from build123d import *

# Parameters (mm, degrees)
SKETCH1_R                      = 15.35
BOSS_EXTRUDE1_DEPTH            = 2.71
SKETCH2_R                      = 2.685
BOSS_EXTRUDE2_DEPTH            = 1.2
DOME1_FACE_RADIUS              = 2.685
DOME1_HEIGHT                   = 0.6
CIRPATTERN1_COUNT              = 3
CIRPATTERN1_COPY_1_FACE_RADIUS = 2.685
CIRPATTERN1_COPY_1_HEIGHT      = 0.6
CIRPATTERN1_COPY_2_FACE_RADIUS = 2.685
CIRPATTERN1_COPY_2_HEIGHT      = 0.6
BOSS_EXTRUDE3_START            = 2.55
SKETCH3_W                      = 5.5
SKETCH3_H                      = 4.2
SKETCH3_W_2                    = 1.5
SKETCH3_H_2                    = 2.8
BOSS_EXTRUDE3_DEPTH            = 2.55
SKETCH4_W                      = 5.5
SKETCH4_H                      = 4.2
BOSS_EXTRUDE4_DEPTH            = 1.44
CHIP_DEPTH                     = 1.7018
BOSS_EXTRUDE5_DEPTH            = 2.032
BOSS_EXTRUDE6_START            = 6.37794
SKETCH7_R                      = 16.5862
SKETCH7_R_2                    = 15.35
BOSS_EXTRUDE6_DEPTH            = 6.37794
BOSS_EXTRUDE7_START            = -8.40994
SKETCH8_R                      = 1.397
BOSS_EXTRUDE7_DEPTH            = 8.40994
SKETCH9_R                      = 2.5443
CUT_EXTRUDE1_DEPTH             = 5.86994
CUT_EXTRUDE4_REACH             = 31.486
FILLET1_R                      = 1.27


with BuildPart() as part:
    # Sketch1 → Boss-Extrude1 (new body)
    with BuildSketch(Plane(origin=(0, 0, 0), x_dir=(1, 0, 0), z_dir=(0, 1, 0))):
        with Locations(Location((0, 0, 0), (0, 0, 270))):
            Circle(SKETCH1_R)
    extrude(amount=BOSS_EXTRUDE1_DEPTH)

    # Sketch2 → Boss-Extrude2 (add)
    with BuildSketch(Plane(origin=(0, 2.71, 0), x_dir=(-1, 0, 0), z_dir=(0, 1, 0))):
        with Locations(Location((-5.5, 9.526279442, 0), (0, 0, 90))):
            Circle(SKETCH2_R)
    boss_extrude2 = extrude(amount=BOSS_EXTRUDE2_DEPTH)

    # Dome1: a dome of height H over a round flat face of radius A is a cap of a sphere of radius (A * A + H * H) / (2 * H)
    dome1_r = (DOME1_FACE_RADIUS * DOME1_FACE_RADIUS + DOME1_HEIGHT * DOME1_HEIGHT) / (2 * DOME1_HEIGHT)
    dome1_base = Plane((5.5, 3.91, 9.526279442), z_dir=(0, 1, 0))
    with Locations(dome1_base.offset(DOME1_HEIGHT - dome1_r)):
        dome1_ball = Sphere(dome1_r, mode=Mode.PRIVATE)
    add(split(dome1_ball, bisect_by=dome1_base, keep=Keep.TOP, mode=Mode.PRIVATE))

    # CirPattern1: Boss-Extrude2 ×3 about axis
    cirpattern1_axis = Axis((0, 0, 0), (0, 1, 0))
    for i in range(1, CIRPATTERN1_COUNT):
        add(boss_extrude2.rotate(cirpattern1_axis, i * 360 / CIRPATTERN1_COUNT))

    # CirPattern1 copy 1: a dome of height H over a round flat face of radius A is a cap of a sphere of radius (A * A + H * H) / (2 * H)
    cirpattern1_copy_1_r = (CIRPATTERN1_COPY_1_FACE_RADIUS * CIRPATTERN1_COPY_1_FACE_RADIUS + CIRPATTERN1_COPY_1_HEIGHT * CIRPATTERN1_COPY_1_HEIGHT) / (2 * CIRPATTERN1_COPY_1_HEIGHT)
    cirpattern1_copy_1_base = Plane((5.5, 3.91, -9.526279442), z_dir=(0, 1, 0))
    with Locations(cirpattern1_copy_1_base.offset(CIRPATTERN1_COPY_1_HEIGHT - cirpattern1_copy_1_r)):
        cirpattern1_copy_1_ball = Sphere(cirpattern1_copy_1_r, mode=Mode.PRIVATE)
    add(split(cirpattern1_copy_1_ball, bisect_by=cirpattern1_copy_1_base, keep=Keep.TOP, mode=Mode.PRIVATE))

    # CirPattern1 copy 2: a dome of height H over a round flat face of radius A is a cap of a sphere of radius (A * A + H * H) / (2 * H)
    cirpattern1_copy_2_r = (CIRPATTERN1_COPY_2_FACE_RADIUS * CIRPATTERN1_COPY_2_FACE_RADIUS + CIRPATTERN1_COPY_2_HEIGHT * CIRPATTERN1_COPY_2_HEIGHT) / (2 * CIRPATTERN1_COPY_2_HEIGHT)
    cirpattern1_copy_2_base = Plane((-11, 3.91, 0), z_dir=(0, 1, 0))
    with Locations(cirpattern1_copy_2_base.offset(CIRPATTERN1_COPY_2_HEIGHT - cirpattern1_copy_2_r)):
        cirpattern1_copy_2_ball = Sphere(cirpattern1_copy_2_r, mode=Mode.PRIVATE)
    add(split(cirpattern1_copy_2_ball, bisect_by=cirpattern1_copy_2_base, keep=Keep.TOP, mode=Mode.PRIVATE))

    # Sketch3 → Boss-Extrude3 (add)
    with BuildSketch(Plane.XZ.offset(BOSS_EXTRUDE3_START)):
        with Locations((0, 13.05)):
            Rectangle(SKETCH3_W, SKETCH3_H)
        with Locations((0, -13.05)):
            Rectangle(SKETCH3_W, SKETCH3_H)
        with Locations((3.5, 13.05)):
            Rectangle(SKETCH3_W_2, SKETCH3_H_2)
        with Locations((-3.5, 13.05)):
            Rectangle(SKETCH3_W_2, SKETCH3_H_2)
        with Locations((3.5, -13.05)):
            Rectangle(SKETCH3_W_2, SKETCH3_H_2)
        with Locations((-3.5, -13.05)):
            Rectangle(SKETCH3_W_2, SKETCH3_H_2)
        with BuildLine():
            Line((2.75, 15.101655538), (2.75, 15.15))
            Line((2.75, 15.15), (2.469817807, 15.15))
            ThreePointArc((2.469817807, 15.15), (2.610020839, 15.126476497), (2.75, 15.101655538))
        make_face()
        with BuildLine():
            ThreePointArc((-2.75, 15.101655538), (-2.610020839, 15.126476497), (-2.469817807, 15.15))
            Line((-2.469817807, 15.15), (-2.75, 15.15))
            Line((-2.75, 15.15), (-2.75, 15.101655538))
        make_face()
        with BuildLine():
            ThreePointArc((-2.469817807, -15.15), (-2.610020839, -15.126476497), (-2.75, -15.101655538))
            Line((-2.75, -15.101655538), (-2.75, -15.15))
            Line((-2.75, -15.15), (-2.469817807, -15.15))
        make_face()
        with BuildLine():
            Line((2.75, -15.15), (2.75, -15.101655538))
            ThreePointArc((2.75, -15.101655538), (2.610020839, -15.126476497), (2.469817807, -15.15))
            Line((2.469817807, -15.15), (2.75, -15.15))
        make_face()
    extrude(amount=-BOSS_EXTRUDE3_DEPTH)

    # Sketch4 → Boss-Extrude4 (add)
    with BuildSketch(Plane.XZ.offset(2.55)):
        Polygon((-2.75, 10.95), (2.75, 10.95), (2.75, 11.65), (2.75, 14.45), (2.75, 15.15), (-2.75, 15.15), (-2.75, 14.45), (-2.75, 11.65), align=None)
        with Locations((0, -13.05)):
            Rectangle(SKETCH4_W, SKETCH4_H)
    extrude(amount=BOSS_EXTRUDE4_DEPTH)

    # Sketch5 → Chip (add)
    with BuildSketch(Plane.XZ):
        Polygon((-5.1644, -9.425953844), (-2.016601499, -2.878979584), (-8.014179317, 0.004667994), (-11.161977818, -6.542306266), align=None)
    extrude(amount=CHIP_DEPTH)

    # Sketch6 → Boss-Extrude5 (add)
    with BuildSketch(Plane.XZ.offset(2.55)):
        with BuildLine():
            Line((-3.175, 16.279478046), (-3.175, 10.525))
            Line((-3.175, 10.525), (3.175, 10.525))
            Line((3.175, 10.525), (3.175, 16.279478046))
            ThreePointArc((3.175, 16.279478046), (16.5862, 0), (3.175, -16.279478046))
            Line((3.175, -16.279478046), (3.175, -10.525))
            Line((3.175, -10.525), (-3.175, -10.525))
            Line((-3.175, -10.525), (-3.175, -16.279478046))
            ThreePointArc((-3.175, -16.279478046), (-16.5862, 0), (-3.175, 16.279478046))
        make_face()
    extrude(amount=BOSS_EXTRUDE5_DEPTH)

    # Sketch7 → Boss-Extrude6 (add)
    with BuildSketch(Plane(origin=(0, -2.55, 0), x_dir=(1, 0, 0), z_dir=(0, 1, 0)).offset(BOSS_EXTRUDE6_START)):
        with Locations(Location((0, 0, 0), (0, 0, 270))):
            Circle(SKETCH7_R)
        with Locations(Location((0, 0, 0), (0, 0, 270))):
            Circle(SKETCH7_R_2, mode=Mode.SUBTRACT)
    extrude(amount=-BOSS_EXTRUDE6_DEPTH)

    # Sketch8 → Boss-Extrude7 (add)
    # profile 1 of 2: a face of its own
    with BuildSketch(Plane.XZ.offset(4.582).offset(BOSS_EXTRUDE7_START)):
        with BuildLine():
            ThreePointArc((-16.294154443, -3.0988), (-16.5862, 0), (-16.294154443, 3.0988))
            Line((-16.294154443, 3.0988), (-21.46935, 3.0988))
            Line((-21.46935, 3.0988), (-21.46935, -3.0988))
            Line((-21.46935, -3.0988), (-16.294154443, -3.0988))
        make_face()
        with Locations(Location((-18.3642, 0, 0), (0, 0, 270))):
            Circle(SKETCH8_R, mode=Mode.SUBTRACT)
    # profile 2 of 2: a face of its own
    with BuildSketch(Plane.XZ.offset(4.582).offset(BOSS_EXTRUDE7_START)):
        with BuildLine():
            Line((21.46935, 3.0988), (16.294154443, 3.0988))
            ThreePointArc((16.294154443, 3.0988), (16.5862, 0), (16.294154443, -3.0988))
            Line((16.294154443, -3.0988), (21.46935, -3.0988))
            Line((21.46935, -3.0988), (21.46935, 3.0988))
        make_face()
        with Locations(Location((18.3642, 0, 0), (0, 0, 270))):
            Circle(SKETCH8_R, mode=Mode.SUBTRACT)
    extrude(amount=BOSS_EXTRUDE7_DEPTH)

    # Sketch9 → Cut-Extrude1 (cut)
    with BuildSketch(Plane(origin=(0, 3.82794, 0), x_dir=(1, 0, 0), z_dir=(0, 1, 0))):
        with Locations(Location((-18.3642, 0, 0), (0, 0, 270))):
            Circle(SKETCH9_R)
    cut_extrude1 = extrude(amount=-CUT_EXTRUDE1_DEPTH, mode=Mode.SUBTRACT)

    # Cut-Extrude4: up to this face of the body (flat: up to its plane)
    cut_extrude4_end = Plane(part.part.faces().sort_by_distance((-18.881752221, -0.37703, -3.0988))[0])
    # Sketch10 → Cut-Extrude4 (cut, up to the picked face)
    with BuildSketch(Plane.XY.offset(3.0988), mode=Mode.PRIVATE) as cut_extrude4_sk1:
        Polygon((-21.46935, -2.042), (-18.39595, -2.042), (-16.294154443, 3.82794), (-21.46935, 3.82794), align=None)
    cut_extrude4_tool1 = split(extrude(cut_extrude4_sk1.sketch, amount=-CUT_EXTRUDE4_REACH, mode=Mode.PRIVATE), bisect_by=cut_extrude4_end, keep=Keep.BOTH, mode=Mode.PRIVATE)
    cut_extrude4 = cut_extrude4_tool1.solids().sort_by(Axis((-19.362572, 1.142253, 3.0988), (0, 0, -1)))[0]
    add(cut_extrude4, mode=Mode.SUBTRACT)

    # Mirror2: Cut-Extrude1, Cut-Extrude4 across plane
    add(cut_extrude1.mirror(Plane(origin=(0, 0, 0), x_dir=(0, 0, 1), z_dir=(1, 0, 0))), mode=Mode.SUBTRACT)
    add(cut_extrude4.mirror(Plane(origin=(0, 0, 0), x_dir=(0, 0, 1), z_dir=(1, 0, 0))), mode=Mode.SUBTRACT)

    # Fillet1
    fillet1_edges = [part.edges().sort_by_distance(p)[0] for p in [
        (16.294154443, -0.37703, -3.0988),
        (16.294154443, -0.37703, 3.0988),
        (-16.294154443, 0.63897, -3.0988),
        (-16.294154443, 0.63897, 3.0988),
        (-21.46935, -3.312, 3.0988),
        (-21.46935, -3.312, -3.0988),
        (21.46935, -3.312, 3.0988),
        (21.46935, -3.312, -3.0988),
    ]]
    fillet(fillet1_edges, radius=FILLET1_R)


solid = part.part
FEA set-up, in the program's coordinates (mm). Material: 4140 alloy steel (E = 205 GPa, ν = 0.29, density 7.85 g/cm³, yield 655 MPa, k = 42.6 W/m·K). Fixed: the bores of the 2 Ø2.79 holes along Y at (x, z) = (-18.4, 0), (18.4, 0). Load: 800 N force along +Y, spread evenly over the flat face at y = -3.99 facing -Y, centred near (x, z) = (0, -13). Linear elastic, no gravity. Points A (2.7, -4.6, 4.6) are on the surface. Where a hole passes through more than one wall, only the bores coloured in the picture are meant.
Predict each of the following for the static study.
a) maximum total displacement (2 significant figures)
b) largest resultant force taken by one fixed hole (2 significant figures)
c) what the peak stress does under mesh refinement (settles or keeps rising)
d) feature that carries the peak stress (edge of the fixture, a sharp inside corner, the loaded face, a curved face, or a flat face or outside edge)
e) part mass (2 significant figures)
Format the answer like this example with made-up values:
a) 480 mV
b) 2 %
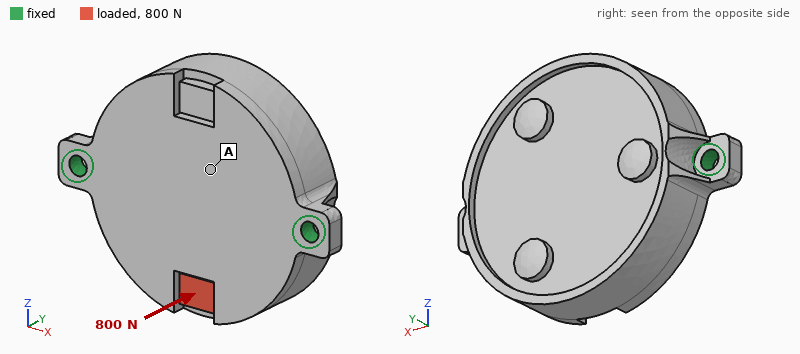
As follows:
a) 84 µm
b) 500 N
c) keeps rising
d) edge of the fixture
e) 39 g
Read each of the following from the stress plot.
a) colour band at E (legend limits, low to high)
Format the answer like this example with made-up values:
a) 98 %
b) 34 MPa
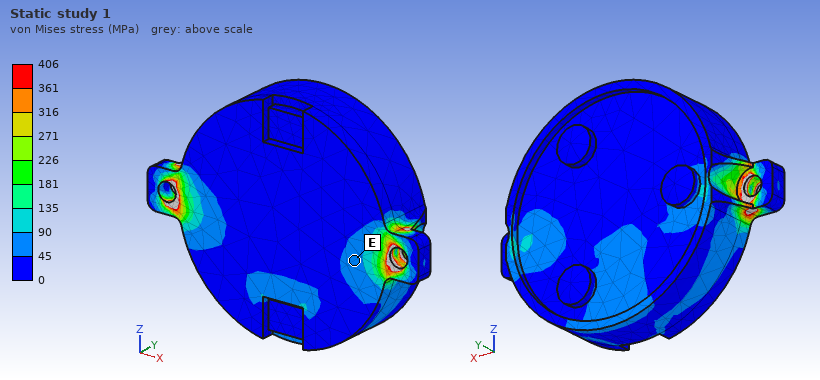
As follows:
a) 45 to 90 MPa
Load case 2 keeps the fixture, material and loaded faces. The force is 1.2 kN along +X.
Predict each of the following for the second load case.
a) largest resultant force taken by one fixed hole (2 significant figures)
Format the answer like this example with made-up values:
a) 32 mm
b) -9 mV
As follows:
a) 750 N
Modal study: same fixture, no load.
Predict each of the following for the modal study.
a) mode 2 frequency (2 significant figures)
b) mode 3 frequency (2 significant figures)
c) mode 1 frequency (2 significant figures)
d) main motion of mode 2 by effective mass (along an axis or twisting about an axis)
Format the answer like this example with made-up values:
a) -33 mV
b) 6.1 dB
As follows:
a) 9600 Hz
b) 18 kHz
c) 4500 Hz
d) along Y
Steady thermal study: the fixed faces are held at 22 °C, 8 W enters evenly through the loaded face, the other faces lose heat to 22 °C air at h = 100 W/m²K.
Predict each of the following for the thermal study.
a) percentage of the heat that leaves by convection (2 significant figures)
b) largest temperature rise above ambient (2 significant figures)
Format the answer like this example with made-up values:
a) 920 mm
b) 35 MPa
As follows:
a) 64 %
b) 55 K
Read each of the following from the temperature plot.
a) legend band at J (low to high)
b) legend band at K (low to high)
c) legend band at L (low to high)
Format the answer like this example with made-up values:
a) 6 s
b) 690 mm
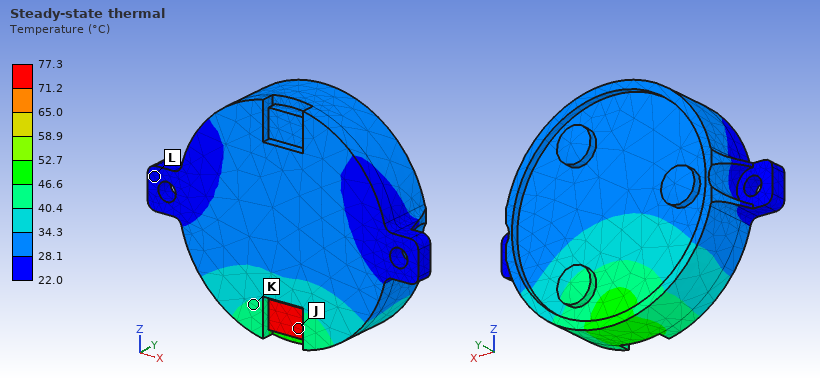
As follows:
a) 71.2 to 77.3 °C
b) 40.4 to 46.6 °C
c) 22.0 to 28.1 °C
